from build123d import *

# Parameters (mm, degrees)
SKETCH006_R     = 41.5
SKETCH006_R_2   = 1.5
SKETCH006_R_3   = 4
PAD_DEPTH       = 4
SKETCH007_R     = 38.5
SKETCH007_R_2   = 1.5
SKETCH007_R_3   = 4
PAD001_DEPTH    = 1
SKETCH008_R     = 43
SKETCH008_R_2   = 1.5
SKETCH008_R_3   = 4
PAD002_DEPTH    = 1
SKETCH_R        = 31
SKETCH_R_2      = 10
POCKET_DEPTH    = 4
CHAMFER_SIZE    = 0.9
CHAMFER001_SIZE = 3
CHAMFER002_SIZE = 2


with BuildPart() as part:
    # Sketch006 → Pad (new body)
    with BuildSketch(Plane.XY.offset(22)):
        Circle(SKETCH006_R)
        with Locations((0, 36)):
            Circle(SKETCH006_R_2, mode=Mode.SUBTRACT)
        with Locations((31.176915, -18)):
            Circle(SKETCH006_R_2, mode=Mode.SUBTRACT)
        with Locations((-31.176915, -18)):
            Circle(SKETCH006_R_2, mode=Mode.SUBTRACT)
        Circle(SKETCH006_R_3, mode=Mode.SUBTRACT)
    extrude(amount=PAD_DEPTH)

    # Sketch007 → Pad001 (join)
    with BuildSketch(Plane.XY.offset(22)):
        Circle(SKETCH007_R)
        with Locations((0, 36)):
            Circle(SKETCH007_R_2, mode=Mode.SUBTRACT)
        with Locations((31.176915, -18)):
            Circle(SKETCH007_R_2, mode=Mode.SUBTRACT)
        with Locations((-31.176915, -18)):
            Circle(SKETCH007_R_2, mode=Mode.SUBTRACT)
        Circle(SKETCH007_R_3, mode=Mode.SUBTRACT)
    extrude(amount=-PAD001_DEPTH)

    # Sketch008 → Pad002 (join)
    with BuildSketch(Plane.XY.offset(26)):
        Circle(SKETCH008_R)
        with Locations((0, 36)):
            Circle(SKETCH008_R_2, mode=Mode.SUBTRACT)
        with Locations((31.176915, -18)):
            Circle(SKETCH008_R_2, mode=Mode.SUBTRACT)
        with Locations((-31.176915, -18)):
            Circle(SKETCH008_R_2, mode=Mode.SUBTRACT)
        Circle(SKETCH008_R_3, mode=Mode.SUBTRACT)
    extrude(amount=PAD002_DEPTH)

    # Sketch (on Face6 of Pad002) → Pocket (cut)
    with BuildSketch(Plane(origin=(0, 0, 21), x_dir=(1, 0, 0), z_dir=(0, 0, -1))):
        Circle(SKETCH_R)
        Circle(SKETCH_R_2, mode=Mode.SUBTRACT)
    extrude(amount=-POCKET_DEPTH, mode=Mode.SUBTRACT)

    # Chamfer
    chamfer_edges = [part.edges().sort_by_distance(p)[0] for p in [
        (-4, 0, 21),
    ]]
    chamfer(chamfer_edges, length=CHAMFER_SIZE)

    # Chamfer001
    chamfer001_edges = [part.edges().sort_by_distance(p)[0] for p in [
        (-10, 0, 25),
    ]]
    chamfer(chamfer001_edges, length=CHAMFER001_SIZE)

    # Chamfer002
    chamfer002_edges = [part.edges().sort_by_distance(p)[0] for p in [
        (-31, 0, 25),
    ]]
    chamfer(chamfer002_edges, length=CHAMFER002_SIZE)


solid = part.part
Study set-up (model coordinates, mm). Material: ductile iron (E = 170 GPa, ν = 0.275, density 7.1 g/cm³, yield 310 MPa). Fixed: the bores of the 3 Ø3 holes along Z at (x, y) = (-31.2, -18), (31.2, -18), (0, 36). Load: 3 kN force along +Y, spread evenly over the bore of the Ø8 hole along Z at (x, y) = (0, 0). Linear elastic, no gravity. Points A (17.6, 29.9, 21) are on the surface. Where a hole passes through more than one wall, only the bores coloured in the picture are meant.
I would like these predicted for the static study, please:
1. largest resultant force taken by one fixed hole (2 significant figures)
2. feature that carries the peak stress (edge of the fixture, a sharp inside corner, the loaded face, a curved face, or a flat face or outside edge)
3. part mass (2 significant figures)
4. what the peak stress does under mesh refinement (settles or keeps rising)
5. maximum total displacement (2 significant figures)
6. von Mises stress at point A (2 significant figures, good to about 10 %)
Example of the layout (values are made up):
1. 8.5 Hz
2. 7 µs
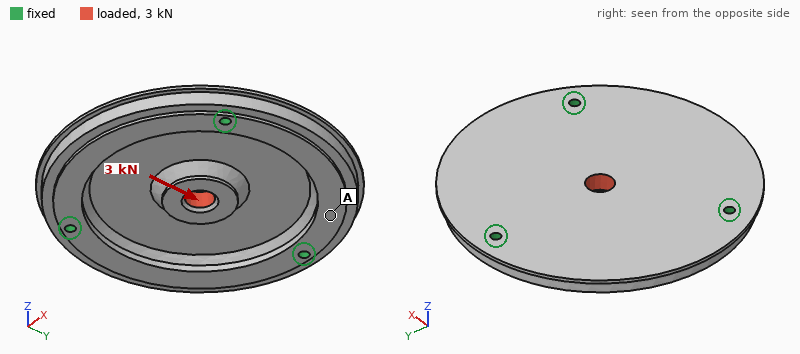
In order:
1. 1.0 kN
2. edge of the fixture
3. 150 g
4. keeps rising
5. 12 µm
6. 4.6 MPa
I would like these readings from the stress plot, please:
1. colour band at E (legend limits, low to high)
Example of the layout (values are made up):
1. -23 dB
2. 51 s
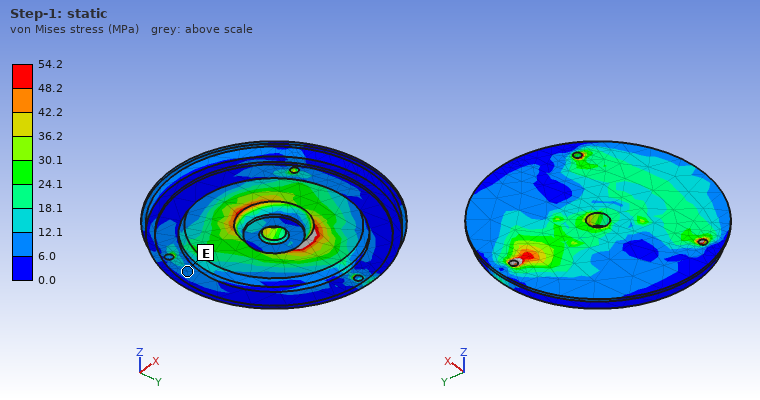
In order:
1. 6.0 to 12.1 MPa
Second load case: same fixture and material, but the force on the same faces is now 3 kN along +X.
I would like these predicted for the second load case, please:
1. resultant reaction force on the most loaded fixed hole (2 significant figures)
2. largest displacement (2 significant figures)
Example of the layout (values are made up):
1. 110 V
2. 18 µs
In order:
1. 1.0 kN
2. 12 µm
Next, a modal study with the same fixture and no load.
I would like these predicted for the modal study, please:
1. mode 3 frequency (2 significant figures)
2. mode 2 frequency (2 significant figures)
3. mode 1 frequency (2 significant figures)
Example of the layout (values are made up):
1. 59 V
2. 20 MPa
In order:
1. 4400 Hz
2. 4400 Hz
3. 4300 Hz
